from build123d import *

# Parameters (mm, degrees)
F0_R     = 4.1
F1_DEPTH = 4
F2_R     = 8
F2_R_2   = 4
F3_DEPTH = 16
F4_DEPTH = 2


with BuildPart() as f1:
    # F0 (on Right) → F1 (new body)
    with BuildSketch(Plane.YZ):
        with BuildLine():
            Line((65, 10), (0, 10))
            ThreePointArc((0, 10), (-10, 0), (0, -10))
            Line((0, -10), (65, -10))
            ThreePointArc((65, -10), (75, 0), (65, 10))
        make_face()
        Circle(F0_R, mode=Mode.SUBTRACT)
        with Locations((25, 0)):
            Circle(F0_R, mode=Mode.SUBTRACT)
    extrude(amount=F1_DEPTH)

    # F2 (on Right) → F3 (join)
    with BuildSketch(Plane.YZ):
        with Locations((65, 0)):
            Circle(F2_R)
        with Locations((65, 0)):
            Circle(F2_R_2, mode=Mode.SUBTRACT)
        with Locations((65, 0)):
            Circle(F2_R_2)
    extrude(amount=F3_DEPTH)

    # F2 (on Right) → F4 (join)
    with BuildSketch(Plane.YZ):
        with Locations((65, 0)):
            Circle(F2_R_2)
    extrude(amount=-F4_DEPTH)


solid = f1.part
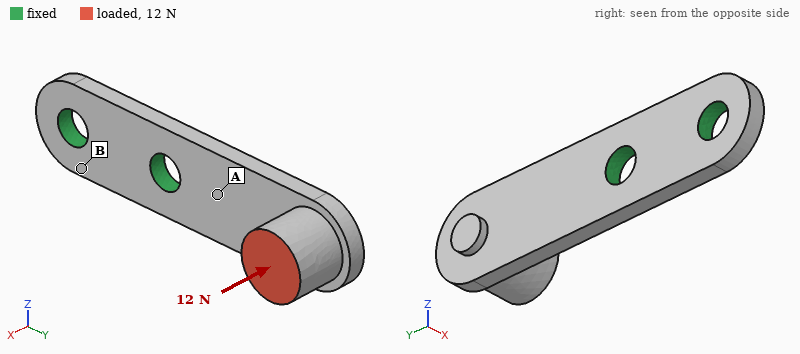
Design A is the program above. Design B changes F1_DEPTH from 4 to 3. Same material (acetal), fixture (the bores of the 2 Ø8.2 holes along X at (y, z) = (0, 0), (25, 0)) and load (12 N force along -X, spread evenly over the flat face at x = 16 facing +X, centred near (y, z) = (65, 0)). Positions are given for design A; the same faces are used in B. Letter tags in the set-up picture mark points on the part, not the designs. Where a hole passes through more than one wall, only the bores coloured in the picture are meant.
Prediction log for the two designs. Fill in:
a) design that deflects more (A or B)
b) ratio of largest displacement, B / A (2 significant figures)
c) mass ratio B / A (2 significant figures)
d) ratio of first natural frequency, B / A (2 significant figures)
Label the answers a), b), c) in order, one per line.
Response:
a) B
b) 2.3
c) 0.85
d) 0.67
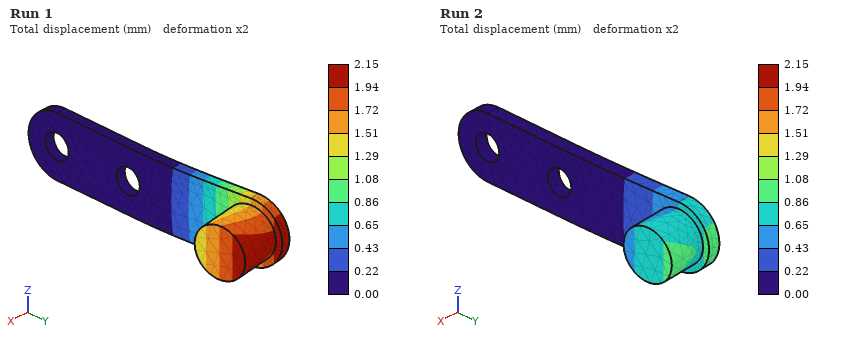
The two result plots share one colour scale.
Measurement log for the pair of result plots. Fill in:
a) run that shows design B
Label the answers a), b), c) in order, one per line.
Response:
a) Run 1
